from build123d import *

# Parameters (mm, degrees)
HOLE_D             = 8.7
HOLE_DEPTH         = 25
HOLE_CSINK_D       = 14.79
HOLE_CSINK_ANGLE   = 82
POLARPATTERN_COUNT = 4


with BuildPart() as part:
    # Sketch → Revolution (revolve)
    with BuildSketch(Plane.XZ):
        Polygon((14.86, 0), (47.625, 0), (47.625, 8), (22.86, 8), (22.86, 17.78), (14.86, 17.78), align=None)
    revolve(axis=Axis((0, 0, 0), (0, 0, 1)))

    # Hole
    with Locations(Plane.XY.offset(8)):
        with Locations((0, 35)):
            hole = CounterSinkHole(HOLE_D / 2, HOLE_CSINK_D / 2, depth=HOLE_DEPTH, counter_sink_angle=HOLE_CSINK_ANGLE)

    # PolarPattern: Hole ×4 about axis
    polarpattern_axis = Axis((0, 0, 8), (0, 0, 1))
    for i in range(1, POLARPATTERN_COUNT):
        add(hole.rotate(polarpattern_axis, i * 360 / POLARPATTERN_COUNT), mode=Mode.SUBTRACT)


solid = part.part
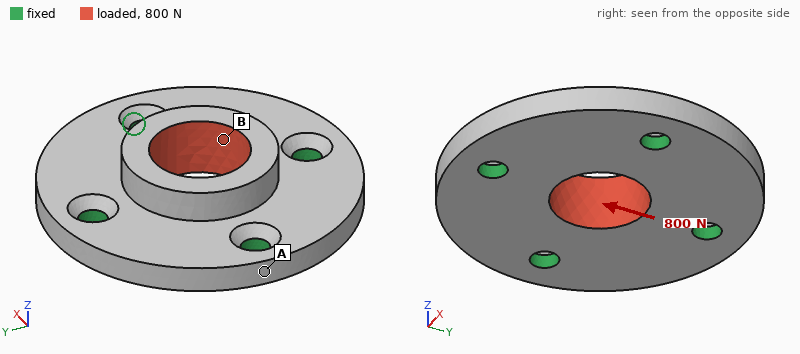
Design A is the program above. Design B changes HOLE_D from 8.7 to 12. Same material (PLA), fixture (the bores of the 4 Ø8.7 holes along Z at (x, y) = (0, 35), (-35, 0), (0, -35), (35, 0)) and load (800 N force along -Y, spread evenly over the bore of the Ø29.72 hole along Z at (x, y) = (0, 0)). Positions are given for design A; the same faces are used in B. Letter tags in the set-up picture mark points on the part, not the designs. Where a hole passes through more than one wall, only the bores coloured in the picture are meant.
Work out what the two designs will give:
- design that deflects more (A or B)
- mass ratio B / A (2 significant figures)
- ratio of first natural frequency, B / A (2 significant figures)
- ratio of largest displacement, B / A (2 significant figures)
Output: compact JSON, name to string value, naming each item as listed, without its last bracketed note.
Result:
{"design that deflects more": "A", "mass ratio B / A": "0.98", "ratio of first natural frequency, B / A": "1.3", "ratio of largest displacement, B / A": "0.85"}
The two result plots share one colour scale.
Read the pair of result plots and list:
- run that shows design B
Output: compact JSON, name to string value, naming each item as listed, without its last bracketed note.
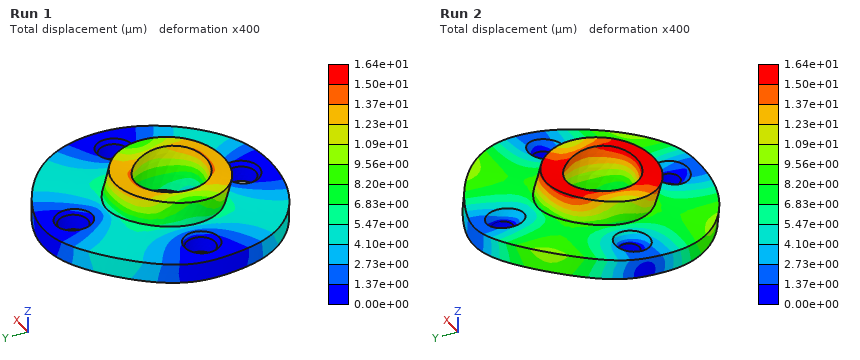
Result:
{"run that shows design B": "Run 1"}
